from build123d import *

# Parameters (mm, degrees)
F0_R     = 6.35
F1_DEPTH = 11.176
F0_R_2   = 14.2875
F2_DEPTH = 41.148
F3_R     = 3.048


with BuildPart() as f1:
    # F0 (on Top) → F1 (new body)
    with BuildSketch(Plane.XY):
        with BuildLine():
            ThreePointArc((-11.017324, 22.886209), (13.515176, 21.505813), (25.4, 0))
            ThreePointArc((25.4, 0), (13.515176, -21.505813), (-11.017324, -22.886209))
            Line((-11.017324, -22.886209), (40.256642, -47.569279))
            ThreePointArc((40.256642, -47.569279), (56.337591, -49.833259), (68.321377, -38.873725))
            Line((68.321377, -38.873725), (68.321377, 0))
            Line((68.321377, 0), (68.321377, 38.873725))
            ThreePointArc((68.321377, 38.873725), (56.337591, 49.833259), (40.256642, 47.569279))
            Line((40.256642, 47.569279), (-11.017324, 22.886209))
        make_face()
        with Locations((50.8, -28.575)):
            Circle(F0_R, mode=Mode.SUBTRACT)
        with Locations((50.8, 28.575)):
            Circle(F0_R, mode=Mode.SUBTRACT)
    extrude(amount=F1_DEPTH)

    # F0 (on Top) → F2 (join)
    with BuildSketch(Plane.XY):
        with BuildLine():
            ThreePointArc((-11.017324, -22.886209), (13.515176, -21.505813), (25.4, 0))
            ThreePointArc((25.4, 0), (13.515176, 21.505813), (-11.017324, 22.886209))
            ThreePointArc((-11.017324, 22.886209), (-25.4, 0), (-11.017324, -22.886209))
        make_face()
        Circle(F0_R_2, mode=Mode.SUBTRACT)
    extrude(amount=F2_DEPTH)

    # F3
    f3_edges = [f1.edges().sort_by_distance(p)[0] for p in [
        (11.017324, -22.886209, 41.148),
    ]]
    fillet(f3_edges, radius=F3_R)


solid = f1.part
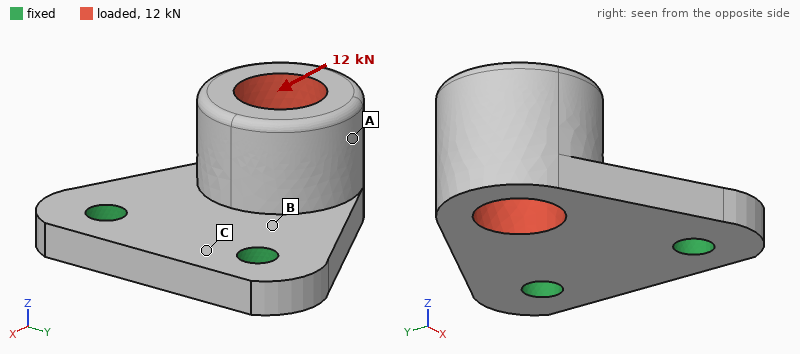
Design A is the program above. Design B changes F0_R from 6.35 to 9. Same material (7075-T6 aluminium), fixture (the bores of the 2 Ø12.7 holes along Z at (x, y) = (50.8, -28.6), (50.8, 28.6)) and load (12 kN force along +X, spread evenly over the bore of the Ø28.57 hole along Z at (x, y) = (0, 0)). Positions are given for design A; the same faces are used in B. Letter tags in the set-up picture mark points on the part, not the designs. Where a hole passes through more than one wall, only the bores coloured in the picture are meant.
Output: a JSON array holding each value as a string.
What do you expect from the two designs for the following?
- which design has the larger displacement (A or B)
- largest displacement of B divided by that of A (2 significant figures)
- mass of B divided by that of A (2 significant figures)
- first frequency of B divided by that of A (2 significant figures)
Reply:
["A", "0.89", "0.97", "1.1"]
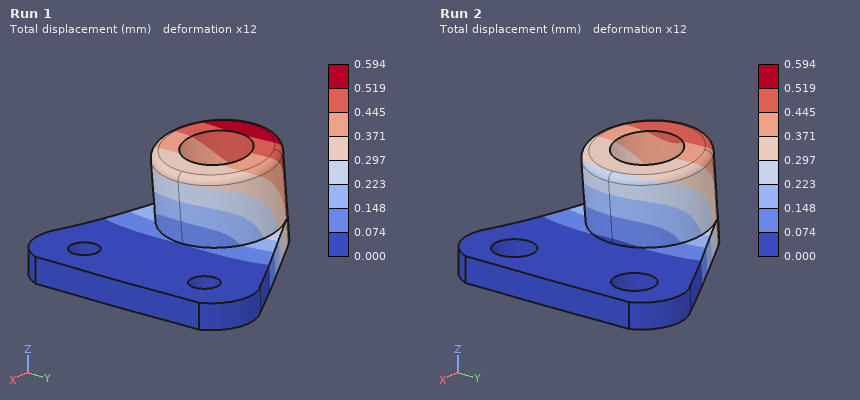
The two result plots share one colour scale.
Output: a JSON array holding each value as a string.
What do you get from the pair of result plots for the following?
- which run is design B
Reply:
["Run 2"]
